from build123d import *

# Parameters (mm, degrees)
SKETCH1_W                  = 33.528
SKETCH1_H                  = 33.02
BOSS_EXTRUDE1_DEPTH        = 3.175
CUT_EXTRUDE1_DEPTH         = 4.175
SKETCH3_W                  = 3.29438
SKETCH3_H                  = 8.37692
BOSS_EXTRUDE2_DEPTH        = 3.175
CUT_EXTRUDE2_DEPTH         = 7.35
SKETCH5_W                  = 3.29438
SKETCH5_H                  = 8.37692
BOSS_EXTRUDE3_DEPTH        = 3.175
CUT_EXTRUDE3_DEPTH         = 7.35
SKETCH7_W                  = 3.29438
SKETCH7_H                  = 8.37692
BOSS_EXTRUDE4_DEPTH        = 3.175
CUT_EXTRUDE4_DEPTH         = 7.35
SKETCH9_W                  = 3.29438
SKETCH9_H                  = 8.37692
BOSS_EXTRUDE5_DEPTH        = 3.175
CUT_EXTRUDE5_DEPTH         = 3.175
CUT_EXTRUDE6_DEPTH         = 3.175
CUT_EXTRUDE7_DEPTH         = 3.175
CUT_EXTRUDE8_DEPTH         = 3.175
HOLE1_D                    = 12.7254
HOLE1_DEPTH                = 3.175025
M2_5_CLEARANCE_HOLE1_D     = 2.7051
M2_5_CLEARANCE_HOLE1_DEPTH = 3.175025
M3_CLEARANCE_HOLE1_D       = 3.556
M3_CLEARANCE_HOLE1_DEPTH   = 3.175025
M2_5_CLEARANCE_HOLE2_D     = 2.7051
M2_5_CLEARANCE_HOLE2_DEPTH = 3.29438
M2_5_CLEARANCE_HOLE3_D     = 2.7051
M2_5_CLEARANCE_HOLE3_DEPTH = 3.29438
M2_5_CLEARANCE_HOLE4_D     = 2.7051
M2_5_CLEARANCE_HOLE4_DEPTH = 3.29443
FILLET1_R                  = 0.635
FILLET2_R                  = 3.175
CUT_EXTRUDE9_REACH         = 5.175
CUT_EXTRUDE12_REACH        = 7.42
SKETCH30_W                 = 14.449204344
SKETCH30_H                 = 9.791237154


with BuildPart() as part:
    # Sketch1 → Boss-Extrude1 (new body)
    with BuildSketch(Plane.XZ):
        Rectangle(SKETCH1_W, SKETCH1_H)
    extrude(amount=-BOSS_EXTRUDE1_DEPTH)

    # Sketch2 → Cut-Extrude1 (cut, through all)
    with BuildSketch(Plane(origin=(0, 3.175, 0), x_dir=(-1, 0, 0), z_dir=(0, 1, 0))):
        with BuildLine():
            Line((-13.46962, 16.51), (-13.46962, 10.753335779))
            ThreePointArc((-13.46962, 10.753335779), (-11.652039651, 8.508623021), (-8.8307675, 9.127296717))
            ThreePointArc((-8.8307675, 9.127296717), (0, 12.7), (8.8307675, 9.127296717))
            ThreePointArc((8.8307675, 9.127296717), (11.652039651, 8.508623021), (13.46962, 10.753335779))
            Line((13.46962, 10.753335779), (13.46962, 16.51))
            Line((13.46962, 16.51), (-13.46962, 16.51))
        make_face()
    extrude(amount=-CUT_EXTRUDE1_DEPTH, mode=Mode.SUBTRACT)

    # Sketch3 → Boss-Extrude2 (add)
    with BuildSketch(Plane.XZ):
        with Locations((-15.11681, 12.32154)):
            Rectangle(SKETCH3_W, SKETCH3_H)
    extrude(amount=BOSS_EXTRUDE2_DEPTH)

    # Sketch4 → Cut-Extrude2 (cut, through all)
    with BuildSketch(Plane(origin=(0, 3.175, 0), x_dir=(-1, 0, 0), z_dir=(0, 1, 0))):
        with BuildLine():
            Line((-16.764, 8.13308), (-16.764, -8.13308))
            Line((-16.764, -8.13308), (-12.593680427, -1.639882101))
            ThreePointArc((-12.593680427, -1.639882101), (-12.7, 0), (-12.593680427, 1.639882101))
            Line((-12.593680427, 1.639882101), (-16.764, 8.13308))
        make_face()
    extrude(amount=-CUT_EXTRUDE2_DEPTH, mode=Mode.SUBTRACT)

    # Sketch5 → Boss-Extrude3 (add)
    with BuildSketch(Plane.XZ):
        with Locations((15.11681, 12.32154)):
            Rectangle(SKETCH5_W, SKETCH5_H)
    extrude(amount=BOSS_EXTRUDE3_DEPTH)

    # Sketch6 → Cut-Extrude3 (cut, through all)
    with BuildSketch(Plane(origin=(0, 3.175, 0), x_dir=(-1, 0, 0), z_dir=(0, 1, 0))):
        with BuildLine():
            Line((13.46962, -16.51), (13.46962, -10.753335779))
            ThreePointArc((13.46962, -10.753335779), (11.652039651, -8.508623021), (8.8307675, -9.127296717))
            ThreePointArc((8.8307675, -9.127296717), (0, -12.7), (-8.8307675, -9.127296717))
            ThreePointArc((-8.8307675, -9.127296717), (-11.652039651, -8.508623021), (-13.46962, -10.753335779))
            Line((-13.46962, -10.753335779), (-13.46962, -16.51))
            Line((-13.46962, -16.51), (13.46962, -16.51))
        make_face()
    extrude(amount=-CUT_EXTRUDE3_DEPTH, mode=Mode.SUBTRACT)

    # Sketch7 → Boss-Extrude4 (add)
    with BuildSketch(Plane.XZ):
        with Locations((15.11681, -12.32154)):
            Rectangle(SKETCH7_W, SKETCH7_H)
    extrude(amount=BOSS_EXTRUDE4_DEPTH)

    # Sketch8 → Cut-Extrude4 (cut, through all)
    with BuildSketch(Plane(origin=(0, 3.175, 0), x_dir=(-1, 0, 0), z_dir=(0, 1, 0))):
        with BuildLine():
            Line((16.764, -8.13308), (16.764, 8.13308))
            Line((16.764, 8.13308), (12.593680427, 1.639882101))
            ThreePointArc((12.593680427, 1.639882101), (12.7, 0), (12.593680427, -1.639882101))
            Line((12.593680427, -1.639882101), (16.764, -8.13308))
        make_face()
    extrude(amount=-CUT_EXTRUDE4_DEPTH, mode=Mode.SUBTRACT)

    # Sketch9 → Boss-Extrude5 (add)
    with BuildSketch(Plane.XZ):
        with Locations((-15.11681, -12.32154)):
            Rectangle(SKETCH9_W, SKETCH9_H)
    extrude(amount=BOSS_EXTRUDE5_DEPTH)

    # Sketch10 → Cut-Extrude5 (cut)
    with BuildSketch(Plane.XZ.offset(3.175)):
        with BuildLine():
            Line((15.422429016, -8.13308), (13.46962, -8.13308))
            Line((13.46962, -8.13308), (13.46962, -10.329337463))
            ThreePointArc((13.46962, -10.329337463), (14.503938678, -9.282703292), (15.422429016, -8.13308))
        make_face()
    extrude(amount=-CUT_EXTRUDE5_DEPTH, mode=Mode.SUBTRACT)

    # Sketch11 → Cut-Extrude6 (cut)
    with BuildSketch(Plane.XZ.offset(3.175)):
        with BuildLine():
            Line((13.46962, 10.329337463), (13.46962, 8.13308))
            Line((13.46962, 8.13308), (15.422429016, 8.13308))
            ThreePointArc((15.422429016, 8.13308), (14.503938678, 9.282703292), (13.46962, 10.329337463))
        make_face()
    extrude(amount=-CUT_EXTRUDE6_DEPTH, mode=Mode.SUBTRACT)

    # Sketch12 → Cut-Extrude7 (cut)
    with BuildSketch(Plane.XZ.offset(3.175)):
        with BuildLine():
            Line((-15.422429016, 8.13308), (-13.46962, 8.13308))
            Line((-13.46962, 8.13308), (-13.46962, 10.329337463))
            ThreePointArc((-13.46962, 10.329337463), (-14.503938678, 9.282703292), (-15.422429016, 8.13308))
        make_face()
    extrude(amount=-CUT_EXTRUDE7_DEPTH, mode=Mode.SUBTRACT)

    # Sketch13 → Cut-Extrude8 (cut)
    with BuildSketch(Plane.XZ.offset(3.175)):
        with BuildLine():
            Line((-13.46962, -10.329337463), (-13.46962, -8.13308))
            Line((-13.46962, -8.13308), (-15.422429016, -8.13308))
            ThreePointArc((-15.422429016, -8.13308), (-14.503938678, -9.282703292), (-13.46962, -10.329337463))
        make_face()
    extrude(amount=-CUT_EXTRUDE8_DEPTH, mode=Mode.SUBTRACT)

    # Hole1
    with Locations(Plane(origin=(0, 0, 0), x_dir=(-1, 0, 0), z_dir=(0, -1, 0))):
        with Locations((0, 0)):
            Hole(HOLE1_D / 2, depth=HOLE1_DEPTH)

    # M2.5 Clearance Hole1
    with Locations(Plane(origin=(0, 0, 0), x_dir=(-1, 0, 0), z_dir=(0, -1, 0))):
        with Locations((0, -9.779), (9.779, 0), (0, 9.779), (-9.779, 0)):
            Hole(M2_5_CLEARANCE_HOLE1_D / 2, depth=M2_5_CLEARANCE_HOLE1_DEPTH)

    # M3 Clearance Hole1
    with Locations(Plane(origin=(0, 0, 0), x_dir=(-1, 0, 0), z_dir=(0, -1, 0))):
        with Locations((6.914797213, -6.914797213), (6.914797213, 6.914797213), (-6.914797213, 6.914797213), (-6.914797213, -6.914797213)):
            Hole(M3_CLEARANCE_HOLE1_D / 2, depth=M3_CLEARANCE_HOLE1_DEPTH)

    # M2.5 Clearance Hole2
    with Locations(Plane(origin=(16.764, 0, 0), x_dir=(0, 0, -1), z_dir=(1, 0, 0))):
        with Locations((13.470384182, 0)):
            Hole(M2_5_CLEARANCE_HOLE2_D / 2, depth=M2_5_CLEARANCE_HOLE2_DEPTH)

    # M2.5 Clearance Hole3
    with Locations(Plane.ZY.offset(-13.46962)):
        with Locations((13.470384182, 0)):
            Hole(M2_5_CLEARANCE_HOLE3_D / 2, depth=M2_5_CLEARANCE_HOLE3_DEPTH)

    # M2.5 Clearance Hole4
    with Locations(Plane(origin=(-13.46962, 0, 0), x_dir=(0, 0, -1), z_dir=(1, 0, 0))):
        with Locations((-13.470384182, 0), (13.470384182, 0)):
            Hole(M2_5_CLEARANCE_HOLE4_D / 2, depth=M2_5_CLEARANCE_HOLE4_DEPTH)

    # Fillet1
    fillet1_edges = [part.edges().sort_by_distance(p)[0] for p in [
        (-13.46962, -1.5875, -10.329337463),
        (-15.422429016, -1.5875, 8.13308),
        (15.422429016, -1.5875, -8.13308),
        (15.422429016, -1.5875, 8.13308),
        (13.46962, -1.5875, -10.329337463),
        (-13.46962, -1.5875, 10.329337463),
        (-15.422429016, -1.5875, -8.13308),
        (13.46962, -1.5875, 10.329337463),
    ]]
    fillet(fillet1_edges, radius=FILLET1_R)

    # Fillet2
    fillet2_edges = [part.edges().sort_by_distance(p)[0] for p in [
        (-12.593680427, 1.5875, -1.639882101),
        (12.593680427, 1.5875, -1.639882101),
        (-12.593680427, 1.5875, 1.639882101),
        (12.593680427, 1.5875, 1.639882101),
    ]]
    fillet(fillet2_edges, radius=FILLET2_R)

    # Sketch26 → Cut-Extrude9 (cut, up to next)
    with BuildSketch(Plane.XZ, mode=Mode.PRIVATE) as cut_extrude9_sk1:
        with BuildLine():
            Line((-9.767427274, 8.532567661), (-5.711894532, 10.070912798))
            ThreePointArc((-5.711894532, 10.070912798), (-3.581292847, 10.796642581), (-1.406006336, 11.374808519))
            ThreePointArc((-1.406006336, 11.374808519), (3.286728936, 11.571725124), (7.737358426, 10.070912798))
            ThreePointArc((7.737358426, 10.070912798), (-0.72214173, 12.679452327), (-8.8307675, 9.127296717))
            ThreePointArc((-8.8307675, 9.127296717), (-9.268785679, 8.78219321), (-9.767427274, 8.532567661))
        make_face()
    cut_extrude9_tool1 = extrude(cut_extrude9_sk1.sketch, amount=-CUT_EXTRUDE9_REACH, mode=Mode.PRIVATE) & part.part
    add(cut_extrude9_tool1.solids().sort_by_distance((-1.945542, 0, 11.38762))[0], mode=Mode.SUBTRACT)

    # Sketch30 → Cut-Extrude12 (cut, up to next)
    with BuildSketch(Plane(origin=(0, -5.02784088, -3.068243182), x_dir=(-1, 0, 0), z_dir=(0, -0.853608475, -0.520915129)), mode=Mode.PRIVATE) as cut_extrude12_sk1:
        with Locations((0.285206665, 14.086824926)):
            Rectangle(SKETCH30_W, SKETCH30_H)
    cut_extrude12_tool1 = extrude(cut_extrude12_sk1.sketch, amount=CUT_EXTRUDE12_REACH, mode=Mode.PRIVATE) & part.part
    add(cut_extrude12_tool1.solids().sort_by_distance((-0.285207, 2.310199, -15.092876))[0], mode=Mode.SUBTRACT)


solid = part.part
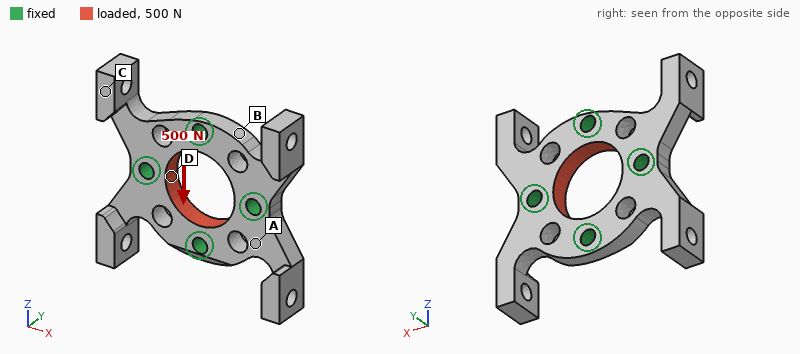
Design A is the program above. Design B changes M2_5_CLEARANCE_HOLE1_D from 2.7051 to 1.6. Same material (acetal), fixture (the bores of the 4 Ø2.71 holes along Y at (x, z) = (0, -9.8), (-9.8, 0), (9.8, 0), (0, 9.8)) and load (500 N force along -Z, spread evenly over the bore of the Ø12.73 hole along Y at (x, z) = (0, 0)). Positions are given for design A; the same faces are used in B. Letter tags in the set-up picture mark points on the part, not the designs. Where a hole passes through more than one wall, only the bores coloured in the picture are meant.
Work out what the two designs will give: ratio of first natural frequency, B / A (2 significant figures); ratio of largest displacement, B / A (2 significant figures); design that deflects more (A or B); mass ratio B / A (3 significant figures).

0.93
1.3
B
1.03
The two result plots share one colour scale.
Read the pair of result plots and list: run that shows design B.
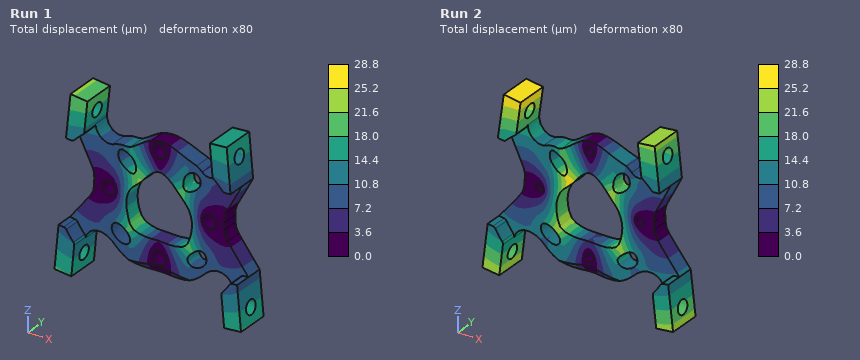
Run 2
